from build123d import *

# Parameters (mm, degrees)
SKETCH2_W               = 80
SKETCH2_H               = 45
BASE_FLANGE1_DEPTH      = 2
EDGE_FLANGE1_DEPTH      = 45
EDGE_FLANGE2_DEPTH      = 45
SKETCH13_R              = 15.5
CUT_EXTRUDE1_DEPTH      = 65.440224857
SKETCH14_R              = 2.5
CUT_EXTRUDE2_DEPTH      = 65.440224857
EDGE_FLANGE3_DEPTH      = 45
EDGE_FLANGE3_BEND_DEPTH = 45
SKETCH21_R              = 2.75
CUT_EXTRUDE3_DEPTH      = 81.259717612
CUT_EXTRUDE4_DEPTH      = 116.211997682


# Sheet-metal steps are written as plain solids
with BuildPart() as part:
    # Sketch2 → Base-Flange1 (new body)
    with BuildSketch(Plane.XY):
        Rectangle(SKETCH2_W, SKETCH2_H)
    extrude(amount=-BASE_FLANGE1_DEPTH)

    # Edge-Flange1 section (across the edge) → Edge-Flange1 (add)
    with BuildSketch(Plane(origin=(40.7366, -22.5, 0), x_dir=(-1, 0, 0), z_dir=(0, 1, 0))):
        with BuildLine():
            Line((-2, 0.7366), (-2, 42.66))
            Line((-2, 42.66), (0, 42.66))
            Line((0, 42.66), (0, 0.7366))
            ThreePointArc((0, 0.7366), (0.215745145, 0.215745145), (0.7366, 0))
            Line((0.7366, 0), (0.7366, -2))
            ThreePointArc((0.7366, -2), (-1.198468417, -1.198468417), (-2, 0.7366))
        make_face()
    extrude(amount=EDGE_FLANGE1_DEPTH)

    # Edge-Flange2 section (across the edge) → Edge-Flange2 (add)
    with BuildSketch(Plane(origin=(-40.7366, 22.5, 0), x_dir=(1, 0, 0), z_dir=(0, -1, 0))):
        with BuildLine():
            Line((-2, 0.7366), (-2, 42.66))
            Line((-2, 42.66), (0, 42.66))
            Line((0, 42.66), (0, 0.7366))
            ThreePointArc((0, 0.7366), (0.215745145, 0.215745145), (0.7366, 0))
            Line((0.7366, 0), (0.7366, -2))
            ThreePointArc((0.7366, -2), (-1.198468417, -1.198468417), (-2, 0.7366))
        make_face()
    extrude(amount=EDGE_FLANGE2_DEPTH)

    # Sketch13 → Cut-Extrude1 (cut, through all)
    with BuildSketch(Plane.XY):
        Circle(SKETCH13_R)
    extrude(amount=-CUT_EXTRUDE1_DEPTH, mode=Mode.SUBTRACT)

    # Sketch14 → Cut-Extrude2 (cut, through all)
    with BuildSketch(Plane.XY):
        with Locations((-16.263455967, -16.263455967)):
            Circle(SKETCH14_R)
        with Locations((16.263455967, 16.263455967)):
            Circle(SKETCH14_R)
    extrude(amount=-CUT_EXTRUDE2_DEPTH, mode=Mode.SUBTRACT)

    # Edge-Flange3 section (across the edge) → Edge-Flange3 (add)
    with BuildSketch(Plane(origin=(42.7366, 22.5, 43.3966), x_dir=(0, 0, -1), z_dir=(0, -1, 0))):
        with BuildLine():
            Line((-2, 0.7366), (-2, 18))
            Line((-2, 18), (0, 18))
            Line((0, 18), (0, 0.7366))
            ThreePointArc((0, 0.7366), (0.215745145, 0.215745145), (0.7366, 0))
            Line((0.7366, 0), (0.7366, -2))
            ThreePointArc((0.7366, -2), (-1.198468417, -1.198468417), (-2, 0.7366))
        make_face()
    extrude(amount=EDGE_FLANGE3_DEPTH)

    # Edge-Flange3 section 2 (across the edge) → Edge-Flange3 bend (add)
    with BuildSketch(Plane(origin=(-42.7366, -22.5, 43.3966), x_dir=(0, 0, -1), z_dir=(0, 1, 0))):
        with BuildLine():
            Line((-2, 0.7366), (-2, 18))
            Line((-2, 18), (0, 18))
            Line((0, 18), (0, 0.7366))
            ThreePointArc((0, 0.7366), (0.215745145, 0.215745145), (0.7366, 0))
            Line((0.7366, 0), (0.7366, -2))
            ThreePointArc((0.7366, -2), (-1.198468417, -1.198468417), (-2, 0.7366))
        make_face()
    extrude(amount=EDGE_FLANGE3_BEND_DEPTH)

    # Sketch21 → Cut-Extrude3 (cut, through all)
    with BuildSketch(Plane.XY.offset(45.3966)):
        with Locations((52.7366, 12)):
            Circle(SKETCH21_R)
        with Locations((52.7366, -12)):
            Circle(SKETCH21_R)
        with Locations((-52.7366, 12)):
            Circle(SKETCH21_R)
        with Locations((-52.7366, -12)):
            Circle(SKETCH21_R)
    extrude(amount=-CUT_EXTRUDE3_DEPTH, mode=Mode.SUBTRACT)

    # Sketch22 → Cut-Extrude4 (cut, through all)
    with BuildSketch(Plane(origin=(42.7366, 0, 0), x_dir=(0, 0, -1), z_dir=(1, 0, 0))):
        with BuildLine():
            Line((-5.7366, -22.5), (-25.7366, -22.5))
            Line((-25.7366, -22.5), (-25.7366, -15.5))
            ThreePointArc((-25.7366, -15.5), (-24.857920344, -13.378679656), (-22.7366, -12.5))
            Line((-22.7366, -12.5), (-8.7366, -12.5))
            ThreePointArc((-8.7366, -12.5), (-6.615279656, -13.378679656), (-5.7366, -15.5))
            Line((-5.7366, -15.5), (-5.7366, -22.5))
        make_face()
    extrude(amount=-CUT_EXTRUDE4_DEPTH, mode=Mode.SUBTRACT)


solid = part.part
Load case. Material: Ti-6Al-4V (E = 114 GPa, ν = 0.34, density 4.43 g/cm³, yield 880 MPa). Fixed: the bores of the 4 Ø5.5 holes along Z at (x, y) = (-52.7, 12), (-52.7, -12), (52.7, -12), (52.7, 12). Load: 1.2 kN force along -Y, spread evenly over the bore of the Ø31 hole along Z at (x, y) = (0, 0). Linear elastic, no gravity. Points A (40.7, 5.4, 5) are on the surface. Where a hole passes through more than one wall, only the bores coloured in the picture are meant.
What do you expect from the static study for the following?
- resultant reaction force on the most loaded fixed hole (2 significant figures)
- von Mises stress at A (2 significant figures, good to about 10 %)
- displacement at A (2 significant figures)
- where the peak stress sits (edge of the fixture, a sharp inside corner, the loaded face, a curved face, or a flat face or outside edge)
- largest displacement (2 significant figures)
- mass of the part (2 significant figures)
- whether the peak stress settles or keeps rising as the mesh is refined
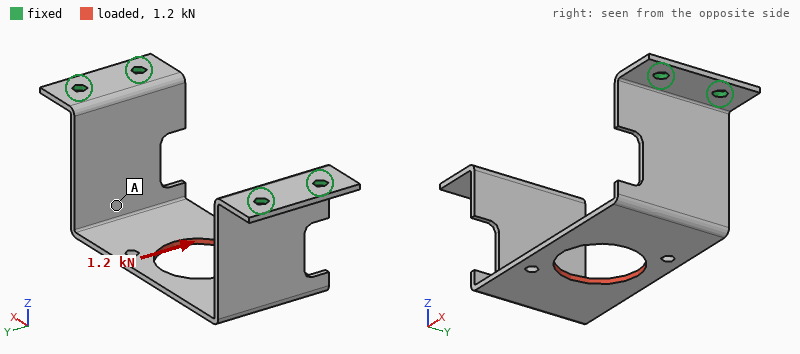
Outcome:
1.1 kN
55 MPa
0.35 mm
edge of the fixture
0.46 mm
72 g
keeps rising
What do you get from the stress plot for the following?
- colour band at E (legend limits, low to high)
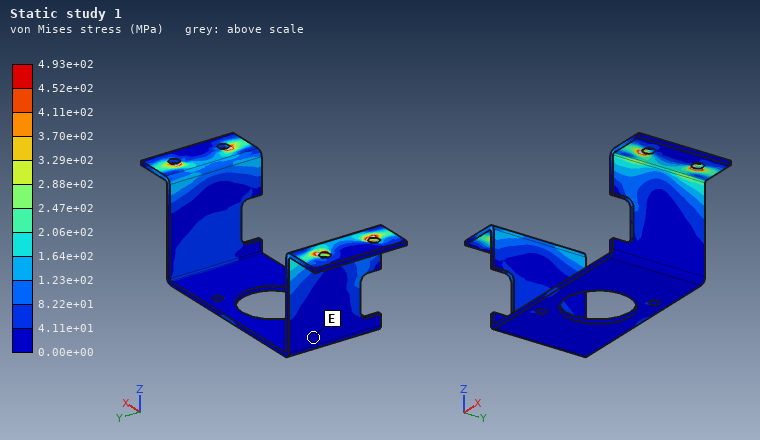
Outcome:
0.00e+00 to 4.11e+01 MPa
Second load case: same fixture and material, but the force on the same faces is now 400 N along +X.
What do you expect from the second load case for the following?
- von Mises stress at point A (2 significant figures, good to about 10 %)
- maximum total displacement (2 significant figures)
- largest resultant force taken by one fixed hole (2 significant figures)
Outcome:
100 MPa
1.1 mm
140 N
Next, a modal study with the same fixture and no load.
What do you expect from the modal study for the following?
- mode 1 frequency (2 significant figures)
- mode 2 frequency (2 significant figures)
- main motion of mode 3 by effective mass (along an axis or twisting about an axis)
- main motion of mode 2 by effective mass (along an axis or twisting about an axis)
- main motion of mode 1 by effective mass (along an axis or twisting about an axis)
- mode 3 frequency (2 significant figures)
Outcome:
510 Hz
1100 Hz
along Y
along Z
along X
1300 Hz
